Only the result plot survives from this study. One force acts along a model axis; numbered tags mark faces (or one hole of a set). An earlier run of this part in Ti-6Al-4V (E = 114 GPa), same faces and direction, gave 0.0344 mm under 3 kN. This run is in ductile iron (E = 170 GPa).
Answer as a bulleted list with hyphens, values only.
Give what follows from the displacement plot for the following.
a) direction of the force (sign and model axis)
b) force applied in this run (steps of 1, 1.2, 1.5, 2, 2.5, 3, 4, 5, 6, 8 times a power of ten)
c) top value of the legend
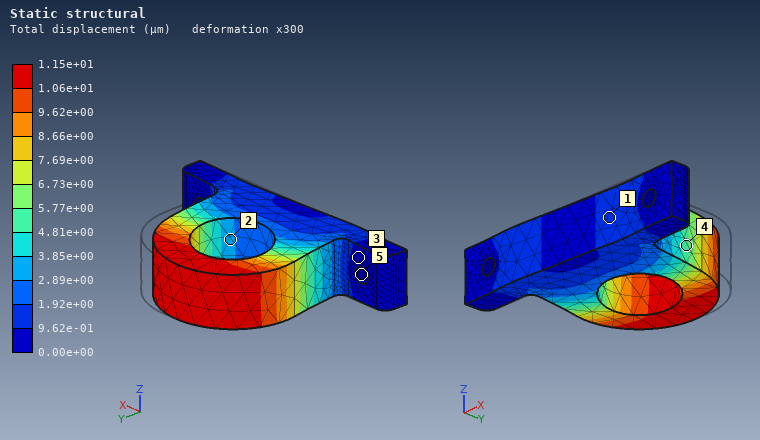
- -X
- 1.5 kN
- 1.15e+01 µm
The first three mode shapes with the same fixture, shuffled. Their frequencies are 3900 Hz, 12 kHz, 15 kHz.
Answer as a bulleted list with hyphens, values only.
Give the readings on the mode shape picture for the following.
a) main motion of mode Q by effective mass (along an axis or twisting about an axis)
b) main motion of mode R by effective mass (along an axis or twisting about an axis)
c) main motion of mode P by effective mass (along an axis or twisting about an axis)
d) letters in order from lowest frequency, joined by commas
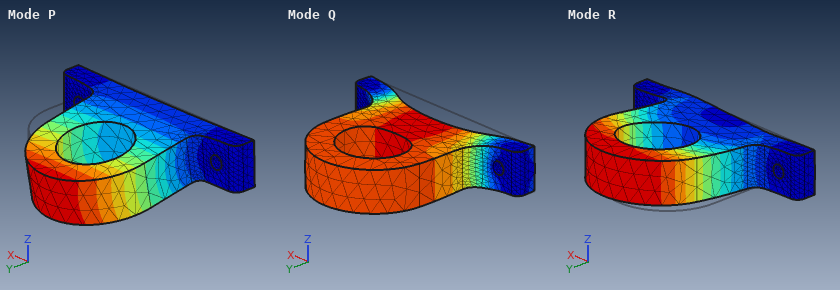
- along Y
- along X
- along Z
- P, R, Q
